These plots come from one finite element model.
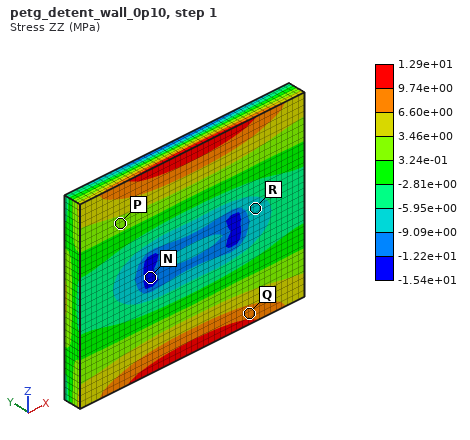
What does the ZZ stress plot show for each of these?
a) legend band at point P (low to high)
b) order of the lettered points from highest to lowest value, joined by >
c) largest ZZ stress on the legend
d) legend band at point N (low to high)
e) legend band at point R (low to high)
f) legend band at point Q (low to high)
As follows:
3.24e-01 to 3.46e+00 MPa
Q > P > R > N
1.29e+01 MPa
-1.54e+01 to -1.22e+01 MPa
-9.09e+00 to -5.95e+00 MPa
6.60e+00 to 9.74e+00 MPa
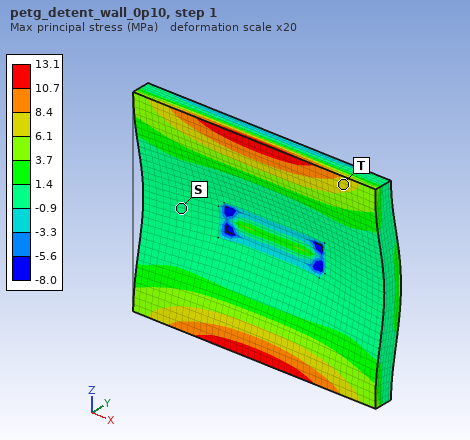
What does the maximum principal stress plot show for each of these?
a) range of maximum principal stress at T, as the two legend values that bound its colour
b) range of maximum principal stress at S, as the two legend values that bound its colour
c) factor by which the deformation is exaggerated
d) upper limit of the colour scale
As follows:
6.1 to 8.4 MPa
-0.9 to 1.4 MPa
20
13.1 MPa
